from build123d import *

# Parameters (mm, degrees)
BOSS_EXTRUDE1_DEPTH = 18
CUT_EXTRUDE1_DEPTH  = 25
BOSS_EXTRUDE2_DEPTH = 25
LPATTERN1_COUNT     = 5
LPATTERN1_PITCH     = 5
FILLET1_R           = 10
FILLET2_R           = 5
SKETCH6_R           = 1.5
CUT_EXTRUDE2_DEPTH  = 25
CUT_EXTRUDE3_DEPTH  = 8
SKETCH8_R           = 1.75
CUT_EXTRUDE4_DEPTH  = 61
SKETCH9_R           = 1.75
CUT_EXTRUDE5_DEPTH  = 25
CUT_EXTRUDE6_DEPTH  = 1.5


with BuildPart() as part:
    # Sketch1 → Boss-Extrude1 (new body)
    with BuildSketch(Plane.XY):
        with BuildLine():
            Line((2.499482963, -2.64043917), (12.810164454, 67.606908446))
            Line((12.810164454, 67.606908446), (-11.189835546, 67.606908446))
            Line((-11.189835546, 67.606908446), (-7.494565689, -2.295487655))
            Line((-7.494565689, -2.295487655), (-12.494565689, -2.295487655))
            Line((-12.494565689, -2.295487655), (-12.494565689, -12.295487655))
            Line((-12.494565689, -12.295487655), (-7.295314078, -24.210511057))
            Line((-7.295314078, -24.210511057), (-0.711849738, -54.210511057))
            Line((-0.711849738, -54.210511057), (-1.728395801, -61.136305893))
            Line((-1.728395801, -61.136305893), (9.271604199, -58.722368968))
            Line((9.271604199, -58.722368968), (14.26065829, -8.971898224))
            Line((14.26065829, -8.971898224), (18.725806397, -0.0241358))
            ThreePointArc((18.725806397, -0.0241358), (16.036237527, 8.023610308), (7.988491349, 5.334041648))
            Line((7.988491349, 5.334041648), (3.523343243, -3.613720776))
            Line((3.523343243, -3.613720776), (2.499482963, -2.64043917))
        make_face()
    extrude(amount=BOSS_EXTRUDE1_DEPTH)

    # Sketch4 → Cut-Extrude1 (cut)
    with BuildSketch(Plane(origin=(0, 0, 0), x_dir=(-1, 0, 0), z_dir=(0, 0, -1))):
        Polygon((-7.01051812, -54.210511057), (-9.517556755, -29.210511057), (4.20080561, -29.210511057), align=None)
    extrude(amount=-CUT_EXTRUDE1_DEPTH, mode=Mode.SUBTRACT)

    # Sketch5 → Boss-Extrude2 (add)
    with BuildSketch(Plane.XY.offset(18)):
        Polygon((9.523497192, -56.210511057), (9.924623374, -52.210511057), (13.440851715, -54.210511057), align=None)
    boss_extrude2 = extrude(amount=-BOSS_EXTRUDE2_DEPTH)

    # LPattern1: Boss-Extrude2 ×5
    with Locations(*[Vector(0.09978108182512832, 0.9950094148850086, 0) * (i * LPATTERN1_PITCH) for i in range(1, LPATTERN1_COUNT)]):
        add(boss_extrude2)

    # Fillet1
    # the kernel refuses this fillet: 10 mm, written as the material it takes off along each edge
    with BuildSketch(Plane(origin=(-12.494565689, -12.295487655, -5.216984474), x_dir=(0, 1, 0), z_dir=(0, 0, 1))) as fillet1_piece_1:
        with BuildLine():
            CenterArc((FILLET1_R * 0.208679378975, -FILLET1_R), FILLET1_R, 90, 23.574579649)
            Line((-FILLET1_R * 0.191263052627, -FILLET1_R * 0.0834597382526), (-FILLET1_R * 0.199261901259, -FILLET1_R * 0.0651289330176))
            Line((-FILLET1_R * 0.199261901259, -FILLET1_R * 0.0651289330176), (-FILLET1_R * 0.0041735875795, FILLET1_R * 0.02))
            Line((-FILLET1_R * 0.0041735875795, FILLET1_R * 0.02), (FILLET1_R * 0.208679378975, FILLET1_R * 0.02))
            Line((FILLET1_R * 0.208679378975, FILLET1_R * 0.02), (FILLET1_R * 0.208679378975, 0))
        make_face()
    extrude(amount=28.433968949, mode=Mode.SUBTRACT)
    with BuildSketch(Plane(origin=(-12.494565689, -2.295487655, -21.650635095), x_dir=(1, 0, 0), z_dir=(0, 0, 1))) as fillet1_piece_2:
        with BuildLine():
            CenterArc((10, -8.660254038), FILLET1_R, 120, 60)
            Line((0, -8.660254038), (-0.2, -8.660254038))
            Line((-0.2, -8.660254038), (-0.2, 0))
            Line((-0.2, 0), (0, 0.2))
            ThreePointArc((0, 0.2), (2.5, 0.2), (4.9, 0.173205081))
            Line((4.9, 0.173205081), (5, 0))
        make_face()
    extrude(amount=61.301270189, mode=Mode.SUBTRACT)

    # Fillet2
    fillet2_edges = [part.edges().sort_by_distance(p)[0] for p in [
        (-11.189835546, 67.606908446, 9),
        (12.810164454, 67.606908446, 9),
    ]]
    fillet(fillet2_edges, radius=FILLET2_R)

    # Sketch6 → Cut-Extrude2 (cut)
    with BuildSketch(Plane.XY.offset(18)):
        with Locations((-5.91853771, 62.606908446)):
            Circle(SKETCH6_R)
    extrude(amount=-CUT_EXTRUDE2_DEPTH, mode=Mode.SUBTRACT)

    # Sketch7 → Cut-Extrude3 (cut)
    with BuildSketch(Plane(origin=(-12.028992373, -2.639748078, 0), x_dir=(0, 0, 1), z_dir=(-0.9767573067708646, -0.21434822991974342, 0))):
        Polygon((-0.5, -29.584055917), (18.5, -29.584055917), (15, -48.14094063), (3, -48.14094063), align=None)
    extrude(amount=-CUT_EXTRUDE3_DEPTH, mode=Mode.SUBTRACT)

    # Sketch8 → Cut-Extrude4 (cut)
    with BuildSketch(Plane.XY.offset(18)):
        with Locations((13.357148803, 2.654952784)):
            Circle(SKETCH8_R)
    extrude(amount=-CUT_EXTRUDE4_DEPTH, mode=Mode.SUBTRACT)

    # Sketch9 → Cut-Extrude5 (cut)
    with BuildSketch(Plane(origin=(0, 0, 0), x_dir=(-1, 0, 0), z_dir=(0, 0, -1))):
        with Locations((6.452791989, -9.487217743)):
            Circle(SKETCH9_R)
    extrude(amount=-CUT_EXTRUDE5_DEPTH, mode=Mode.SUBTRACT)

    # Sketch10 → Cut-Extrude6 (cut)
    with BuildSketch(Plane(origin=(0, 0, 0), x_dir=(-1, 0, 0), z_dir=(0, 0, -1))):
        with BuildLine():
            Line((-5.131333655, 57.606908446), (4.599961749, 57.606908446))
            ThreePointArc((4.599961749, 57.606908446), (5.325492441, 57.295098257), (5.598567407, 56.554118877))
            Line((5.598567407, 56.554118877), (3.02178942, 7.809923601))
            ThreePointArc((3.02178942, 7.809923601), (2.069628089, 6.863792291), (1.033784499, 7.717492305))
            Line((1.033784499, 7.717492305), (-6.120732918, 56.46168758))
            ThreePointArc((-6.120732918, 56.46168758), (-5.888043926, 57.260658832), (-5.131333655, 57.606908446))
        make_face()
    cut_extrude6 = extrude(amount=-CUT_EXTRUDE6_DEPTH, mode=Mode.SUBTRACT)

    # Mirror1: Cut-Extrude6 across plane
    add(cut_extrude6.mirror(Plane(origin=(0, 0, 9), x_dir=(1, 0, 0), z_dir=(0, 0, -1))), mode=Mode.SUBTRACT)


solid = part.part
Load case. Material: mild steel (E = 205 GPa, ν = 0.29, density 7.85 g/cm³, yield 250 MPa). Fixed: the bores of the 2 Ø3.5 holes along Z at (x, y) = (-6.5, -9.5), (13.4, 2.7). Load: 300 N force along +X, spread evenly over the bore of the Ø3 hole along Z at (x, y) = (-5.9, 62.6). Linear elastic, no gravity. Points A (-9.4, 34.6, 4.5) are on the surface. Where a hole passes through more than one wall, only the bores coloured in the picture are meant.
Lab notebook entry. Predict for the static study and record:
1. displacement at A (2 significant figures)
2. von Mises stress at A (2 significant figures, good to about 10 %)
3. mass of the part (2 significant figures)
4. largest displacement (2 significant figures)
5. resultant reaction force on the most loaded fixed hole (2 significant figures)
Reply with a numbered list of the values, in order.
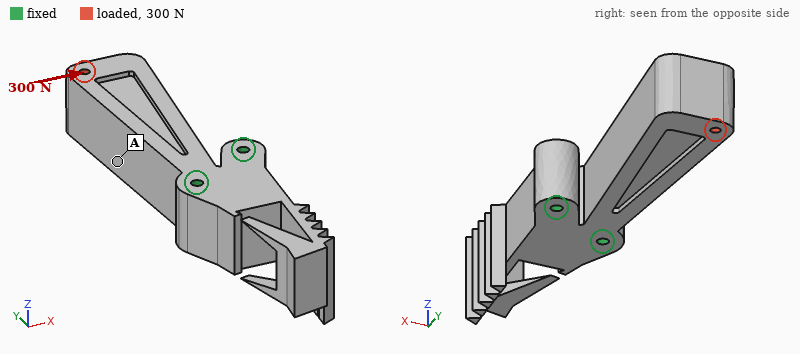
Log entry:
1. 34 µm
2. 9.3 MPa
3. 290 g
4. 72 µm
5. 1.4 kN
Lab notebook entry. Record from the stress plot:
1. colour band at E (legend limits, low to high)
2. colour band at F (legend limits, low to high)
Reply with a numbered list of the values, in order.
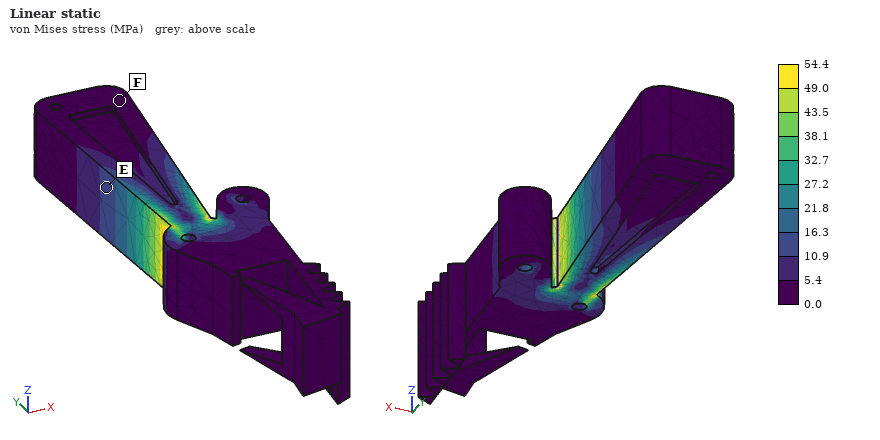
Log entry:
1. 10.9 to 16.3 MPa
2. 0.0 to 5.4 MPa
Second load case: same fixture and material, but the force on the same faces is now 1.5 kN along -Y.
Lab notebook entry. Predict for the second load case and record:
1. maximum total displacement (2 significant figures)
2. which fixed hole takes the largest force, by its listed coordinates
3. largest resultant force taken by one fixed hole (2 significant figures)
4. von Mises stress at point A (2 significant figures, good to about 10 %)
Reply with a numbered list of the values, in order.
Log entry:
1. 24 µm
2. (-6.5, -9.5)
3. 1.4 kN
4. 14 MPa
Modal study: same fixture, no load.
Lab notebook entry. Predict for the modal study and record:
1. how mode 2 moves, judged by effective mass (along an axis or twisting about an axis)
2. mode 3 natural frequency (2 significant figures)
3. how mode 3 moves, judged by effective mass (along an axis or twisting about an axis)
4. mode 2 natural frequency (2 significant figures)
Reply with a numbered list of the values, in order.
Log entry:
1. along X
2. 1900 Hz
3. along Z
4. 1300 Hz
